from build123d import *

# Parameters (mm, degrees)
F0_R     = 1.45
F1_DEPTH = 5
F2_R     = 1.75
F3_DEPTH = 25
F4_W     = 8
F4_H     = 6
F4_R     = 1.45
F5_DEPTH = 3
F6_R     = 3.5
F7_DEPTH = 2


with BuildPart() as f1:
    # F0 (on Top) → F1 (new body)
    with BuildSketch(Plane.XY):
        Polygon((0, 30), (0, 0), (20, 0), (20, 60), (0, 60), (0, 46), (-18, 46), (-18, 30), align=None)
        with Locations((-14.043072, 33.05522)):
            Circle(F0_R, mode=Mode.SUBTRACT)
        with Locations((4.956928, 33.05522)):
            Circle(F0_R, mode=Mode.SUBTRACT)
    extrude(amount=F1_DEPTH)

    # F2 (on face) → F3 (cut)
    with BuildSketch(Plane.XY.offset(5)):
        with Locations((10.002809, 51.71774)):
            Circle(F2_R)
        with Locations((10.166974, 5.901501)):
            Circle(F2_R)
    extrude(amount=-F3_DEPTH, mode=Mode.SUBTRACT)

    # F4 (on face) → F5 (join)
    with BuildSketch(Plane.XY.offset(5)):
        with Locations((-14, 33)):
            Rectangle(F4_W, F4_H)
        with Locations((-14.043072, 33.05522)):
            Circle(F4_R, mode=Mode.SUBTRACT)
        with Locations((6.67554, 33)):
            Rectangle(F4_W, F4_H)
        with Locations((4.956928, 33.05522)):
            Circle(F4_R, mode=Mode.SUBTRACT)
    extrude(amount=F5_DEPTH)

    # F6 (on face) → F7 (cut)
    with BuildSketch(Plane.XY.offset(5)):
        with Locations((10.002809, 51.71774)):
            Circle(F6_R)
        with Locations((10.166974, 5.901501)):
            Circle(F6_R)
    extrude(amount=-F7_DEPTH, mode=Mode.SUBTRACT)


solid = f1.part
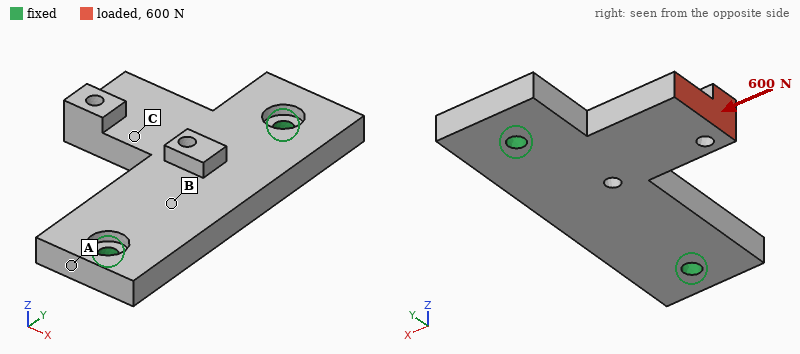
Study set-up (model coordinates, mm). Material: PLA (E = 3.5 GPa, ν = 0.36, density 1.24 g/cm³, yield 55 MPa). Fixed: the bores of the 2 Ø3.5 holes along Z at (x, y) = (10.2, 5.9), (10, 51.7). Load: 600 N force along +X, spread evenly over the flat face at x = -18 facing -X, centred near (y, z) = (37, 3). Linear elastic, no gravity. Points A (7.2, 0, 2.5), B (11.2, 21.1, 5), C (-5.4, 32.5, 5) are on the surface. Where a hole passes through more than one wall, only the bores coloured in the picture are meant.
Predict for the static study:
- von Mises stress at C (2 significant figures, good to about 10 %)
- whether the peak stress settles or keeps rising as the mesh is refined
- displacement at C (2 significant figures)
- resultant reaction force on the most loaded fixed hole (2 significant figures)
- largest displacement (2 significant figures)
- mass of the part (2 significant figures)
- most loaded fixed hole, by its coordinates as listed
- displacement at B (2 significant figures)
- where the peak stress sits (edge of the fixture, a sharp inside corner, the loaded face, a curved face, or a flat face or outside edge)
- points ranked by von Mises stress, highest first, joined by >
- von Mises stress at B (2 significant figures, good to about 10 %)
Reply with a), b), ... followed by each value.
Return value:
a) 17 MPa
b) keeps rising
c) 0.27 mm
d) 410 N
e) 0.60 mm
f) 9.2 g
g) (10, 51.7)
h) 0.099 mm
i) edge of the fixture
j) C > B > A
k) 7.2 MPa
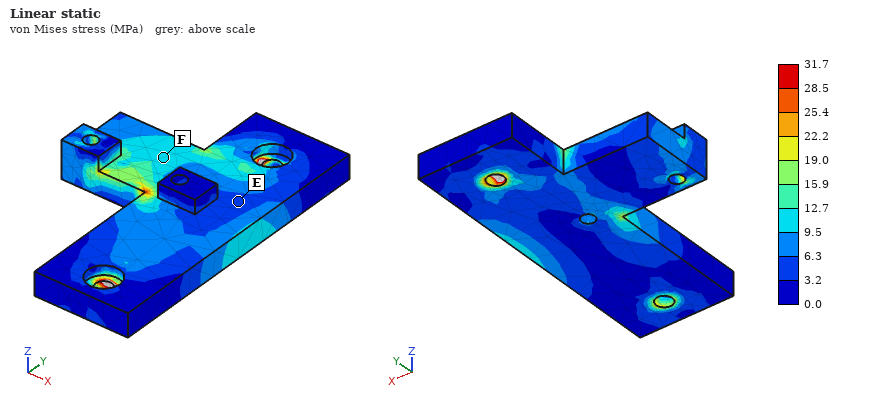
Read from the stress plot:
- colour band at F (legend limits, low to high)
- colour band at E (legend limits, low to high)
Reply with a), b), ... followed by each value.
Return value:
a) 9.5 to 12.7 MPa
b) 3.2 to 6.3 MPa
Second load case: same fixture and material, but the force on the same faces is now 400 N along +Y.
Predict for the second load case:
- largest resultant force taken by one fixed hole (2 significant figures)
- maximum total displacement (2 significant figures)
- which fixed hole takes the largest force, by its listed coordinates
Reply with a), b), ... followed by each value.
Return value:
a) 340 N
b) 0.57 mm
c) (10, 51.7)
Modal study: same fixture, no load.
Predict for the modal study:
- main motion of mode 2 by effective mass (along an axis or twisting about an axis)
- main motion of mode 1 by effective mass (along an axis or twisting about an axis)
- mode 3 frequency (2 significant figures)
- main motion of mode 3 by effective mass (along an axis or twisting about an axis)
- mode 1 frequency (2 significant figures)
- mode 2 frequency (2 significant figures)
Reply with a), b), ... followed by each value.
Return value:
a) along Z
b) along Z
c) 4400 Hz
d) along X
e) 1200 Hz
f) 2900 Hz
